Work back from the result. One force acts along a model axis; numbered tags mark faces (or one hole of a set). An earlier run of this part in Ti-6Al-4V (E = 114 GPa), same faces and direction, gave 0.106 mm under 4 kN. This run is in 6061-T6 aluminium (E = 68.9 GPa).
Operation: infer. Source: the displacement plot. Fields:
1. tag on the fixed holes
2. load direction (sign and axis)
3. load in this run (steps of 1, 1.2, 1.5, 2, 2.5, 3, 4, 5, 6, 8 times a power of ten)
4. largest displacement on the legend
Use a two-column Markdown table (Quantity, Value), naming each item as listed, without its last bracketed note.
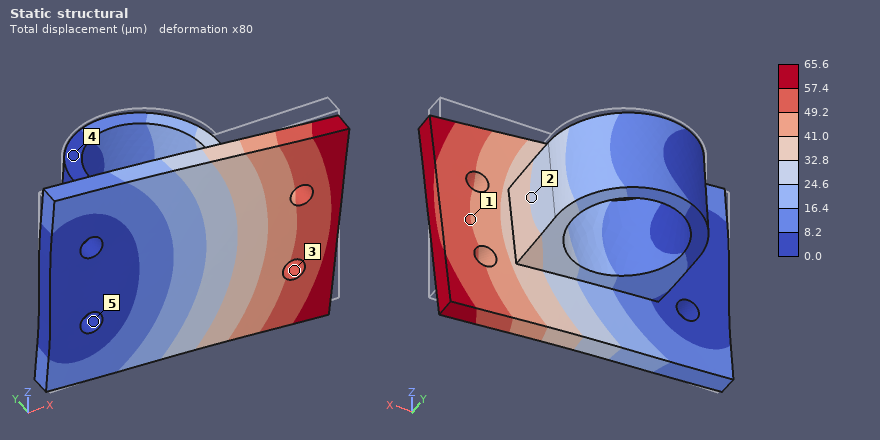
| Quantity | Value |
|---|---|
| tag on the fixed holes | 5 |
| load direction | -Z |
| load in this run | 1.5 kN |
| largest displacement on the legend | 65.6 µm |
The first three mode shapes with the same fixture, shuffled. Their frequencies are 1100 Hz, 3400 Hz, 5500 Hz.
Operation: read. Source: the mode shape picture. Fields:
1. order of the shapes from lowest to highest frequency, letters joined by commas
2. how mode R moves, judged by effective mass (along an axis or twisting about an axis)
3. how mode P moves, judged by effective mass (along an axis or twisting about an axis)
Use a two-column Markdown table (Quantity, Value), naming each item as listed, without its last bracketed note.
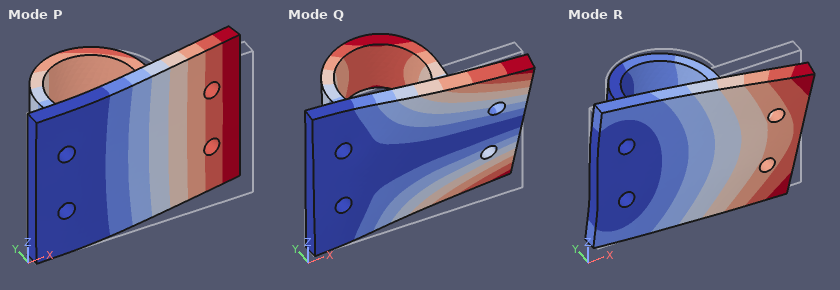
| Quantity | Value |
|---|---|
| order of the shapes from lowest to highest frequency, letters joined by commas | P, Q, R |
| how mode R moves, judged by effective mass | along Z |
| how mode P moves, judged by effective mass | along Y |
